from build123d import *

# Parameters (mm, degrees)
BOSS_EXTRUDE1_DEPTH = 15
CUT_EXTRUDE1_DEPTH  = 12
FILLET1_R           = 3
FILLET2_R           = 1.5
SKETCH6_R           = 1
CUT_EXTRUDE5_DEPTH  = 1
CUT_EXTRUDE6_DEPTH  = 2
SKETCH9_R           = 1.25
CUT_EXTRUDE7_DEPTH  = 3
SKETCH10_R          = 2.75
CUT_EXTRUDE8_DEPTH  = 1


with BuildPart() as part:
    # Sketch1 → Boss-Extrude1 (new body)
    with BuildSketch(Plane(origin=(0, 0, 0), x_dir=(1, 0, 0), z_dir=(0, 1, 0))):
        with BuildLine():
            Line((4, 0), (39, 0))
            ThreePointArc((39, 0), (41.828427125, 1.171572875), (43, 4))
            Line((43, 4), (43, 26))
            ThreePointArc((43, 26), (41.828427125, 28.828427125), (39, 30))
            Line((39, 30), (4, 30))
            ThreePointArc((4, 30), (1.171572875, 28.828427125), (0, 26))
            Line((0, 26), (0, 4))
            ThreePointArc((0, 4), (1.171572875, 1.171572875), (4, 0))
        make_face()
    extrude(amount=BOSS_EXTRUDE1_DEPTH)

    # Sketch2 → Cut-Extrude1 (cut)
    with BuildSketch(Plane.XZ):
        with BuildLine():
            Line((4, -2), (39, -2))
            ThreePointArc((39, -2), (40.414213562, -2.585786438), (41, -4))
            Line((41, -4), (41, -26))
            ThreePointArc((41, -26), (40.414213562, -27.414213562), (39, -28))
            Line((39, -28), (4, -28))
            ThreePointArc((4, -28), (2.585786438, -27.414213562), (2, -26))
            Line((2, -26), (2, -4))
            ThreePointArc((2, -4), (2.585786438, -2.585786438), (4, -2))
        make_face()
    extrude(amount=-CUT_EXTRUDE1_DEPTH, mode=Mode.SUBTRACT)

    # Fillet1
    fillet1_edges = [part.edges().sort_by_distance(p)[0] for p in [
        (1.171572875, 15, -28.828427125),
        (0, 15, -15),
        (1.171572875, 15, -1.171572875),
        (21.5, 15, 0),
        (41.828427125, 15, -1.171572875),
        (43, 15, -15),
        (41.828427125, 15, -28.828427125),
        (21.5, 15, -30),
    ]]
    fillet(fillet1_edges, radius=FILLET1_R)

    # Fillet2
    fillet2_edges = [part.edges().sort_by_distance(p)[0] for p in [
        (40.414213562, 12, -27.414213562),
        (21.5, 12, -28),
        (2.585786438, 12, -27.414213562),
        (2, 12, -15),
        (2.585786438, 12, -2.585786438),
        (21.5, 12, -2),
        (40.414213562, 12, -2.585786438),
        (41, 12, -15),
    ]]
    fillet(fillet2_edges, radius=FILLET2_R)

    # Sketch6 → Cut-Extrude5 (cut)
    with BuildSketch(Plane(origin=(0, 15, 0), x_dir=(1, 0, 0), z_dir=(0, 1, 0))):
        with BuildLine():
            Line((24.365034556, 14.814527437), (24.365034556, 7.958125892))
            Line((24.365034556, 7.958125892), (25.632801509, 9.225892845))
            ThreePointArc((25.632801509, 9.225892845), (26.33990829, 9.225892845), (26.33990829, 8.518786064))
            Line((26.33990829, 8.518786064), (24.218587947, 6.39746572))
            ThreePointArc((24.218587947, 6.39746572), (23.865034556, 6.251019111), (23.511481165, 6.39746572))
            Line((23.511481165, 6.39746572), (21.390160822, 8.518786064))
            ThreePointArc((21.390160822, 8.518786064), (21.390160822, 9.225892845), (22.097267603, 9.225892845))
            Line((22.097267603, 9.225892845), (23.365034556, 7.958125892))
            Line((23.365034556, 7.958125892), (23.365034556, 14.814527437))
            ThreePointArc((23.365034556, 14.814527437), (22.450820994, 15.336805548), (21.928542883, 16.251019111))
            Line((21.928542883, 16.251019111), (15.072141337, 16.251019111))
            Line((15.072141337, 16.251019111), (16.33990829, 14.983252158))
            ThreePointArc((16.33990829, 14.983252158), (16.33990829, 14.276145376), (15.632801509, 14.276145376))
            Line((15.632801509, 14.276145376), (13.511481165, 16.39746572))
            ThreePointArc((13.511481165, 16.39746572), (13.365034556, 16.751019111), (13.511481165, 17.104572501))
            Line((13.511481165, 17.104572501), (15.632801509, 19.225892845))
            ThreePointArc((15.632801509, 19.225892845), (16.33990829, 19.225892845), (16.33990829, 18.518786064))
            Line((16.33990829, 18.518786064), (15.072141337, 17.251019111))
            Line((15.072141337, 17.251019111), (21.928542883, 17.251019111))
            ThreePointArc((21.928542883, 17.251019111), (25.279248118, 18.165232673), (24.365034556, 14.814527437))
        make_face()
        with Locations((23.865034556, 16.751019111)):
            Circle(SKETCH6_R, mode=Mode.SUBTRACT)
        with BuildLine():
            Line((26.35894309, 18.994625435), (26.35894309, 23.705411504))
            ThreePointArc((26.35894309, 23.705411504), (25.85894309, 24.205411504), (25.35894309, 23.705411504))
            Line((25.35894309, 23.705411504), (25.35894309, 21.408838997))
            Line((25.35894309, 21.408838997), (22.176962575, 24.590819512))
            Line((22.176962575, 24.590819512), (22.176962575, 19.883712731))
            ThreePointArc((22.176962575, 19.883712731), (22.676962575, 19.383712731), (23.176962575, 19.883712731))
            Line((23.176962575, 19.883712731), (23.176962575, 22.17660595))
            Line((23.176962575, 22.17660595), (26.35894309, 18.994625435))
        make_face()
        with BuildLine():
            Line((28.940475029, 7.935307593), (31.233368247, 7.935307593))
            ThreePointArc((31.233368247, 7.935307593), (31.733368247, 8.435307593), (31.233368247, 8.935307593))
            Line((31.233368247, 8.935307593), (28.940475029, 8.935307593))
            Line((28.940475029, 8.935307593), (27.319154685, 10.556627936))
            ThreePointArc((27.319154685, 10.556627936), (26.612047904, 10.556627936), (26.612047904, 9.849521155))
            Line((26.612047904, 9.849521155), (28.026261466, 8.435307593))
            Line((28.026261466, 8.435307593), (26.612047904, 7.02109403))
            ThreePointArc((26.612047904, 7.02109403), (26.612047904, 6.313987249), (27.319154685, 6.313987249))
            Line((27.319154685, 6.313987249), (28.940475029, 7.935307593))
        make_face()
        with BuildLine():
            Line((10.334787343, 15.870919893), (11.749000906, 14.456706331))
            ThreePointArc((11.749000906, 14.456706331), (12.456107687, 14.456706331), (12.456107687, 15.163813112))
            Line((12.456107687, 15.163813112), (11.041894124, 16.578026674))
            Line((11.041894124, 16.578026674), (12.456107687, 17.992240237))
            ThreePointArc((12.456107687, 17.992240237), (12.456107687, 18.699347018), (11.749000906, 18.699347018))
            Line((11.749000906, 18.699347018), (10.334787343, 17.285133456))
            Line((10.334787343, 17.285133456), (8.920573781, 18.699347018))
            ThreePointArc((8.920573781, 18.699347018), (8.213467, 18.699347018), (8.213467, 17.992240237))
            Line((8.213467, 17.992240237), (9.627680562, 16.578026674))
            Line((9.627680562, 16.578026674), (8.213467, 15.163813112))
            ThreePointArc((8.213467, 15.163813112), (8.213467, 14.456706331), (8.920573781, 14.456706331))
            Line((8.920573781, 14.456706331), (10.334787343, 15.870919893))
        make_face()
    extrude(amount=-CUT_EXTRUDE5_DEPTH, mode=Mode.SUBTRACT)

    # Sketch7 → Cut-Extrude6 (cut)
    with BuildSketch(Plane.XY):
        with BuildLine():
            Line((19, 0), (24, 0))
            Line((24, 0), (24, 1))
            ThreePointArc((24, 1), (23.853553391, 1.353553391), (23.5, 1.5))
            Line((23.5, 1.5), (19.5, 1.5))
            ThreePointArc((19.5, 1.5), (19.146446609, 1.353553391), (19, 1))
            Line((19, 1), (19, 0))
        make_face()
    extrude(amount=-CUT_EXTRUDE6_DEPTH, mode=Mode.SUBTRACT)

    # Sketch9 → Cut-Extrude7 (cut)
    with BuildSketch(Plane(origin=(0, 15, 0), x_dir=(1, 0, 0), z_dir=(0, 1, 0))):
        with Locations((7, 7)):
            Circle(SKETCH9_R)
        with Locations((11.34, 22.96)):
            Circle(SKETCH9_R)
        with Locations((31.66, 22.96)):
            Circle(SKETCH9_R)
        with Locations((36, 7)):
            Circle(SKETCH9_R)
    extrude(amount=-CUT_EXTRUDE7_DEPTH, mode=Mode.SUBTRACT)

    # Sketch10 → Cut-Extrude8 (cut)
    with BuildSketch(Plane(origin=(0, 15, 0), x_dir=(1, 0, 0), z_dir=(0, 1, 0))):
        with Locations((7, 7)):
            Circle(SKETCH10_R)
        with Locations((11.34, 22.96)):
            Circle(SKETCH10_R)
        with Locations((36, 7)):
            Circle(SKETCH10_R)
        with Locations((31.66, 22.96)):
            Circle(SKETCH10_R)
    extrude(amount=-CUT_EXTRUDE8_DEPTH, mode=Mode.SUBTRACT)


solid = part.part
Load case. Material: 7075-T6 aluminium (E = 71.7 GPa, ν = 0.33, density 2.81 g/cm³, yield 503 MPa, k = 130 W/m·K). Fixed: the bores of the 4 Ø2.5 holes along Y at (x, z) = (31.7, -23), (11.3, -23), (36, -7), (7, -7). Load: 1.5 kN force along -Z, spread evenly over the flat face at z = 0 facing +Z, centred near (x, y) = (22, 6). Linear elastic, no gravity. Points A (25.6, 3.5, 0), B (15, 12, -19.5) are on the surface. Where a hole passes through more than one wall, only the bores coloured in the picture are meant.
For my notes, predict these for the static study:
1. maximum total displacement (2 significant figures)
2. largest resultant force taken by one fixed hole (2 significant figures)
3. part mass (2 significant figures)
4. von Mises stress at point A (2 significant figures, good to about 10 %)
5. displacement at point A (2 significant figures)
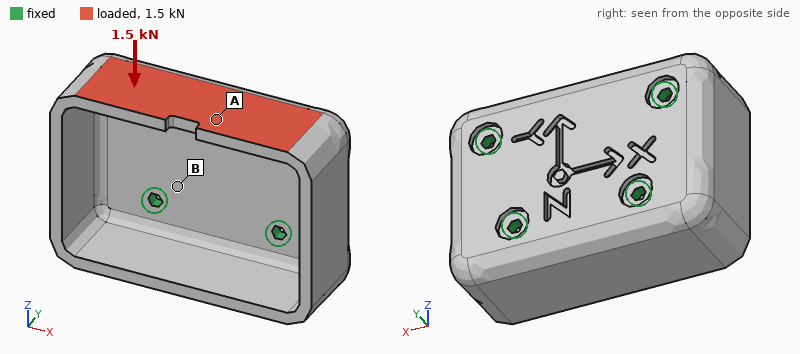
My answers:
0.21 mm
590 N
19 g
69 MPa
0.15 mm
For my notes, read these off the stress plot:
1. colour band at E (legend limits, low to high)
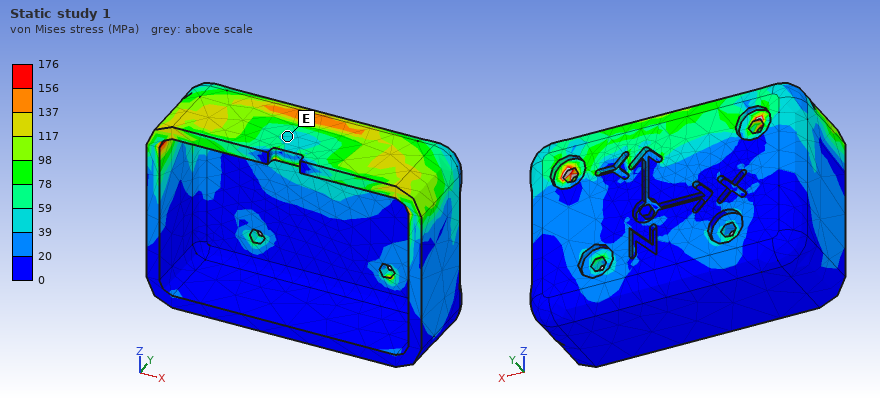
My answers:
39 to 59 MPa
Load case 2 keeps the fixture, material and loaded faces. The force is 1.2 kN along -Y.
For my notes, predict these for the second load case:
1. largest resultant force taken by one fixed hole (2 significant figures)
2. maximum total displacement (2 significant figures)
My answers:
780 N
80 µm
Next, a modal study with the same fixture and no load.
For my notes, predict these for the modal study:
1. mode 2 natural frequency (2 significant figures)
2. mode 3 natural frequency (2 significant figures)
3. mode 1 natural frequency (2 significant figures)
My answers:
10 kHz
11 kHz
10000 Hz
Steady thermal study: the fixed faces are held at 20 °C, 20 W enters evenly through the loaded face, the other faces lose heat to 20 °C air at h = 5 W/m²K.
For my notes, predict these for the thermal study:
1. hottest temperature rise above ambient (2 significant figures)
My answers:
23 K
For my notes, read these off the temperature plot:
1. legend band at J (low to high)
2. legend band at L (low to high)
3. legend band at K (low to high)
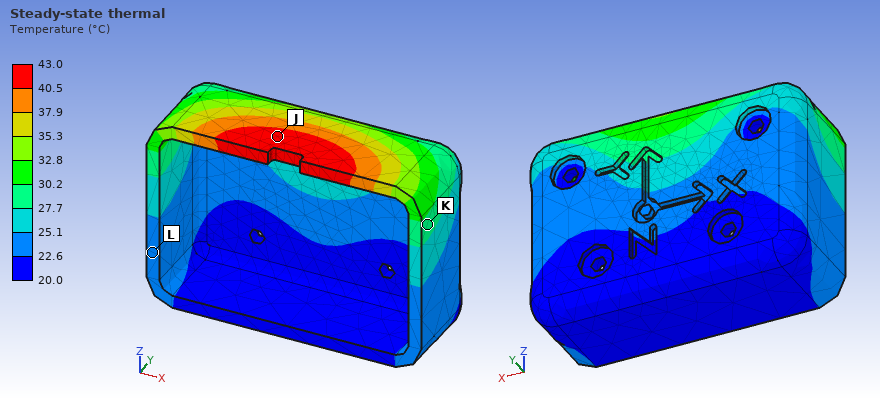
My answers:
40.5 to 43.0 °C
22.6 to 25.1 °C
27.7 to 30.2 °C
